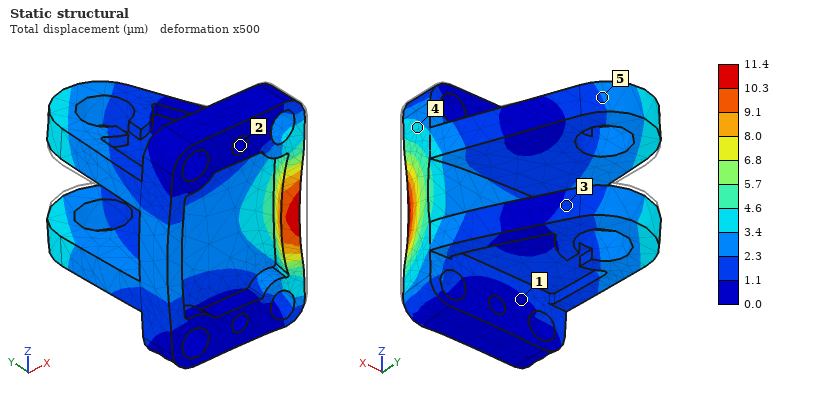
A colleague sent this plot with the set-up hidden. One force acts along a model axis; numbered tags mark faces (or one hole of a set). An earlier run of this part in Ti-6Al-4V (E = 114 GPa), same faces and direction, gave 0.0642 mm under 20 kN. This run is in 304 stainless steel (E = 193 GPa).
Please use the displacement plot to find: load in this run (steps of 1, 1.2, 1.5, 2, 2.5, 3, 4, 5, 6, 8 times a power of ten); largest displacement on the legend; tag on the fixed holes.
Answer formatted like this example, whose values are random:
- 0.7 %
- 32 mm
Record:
- 6 kN
- 11.4 µm
- 2
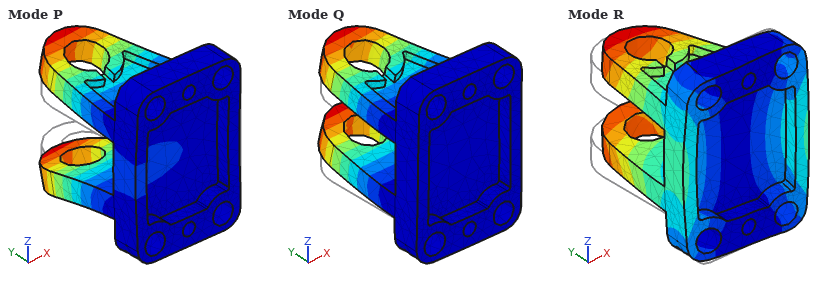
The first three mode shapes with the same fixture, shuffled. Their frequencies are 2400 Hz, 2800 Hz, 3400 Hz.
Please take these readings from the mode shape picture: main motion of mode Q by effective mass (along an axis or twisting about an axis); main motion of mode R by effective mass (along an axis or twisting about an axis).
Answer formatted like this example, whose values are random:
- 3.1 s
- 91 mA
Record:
- along Z
- along X
